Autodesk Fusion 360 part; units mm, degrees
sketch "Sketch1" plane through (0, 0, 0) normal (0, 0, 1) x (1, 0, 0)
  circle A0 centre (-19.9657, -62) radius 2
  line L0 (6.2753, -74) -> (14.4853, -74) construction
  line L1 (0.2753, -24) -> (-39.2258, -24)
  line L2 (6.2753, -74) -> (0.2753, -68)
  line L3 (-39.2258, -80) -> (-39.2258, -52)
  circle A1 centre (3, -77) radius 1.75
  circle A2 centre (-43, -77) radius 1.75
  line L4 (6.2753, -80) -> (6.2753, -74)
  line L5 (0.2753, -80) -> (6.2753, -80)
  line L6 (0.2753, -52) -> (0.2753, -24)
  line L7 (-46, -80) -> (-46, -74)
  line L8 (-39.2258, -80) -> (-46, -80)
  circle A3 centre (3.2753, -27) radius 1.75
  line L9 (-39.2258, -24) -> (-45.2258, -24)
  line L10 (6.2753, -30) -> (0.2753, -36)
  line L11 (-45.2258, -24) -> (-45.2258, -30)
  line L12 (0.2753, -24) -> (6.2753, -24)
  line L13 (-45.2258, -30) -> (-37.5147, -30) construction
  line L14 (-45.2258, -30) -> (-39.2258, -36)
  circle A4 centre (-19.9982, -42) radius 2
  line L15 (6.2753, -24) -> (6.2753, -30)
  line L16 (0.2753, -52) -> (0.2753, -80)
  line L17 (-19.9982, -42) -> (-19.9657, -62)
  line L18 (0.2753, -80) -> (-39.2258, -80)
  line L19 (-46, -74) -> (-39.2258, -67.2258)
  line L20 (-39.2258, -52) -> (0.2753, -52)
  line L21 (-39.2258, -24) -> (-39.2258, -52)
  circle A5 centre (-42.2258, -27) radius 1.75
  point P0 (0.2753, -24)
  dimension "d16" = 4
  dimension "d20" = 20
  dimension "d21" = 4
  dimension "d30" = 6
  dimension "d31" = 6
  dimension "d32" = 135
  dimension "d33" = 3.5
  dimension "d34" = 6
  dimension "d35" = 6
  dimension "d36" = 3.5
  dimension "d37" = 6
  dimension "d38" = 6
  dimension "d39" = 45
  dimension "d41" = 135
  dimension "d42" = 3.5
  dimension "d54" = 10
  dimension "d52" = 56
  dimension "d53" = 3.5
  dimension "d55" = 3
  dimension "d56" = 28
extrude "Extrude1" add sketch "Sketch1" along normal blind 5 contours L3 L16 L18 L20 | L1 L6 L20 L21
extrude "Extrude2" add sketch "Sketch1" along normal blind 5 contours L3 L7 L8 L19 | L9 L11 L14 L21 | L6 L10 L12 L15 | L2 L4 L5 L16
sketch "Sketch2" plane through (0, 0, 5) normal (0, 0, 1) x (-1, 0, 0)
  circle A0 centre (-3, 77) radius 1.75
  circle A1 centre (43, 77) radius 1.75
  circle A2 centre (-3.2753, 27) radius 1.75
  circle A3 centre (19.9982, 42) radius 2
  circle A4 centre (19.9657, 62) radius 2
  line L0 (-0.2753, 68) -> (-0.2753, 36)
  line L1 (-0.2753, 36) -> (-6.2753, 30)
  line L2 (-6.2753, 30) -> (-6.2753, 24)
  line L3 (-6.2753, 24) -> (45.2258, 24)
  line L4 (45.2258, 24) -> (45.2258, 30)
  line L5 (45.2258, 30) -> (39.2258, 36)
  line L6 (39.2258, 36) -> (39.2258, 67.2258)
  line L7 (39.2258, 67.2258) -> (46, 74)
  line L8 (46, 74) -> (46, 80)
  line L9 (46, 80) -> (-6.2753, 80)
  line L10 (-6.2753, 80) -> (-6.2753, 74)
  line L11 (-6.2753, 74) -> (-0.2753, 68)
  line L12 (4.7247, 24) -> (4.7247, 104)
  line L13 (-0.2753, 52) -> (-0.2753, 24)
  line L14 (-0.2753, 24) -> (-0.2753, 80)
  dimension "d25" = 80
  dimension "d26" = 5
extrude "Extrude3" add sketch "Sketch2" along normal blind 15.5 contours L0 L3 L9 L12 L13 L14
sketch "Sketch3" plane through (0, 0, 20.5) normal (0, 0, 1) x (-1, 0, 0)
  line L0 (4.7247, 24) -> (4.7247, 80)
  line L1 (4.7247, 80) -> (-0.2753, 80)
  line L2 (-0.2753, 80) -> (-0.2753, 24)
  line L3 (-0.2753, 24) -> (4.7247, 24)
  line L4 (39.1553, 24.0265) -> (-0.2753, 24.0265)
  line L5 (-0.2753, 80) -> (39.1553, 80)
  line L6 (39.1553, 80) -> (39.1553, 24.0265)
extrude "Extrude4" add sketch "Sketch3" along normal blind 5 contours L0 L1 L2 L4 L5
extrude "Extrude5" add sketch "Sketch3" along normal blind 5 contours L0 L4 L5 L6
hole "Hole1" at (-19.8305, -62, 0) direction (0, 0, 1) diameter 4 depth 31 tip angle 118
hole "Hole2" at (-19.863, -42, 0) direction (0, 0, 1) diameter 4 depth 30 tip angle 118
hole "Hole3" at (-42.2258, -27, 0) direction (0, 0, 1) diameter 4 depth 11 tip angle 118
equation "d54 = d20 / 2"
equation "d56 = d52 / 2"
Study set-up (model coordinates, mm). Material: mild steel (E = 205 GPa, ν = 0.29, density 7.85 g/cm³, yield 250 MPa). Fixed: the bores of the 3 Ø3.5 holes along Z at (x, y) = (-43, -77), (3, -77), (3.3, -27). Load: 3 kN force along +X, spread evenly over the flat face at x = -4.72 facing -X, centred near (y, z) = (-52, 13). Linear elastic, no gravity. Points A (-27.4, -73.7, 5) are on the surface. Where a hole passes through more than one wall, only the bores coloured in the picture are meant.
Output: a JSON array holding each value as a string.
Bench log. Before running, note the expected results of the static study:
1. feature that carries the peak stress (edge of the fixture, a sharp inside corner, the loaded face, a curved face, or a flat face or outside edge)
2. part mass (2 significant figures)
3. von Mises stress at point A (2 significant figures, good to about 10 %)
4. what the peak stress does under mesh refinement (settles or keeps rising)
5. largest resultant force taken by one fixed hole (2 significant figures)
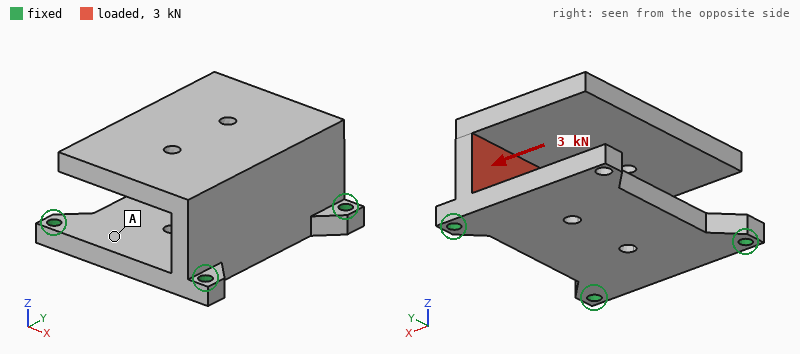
["edge of the fixture", "210 g", "27 MPa", "keeps rising", "1.4 kN"]
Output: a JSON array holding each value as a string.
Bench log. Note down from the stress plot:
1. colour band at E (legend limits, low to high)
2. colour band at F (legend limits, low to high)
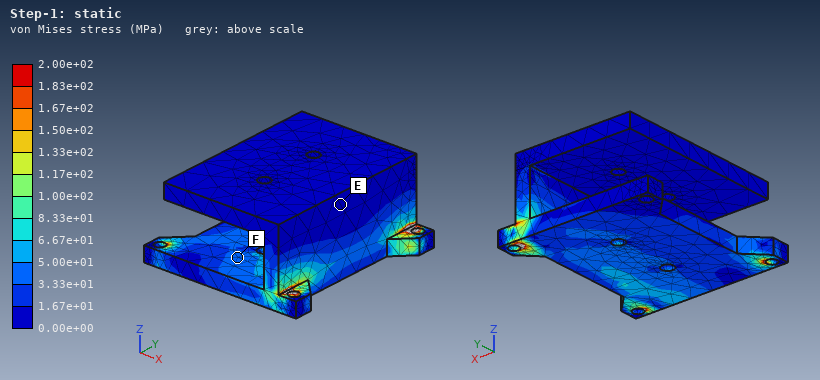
["0.00e+00 to 1.67e+01 MPa", "3.33e+01 to 5.00e+01 MPa"]
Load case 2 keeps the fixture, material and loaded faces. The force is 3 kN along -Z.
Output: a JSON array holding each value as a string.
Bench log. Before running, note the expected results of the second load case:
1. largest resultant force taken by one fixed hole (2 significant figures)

["1.5 kN"]
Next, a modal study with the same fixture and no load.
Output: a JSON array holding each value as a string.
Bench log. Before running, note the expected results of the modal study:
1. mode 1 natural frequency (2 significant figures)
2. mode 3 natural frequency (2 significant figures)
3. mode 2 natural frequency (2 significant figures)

["1300 Hz", "3400 Hz", "2900 Hz"]
